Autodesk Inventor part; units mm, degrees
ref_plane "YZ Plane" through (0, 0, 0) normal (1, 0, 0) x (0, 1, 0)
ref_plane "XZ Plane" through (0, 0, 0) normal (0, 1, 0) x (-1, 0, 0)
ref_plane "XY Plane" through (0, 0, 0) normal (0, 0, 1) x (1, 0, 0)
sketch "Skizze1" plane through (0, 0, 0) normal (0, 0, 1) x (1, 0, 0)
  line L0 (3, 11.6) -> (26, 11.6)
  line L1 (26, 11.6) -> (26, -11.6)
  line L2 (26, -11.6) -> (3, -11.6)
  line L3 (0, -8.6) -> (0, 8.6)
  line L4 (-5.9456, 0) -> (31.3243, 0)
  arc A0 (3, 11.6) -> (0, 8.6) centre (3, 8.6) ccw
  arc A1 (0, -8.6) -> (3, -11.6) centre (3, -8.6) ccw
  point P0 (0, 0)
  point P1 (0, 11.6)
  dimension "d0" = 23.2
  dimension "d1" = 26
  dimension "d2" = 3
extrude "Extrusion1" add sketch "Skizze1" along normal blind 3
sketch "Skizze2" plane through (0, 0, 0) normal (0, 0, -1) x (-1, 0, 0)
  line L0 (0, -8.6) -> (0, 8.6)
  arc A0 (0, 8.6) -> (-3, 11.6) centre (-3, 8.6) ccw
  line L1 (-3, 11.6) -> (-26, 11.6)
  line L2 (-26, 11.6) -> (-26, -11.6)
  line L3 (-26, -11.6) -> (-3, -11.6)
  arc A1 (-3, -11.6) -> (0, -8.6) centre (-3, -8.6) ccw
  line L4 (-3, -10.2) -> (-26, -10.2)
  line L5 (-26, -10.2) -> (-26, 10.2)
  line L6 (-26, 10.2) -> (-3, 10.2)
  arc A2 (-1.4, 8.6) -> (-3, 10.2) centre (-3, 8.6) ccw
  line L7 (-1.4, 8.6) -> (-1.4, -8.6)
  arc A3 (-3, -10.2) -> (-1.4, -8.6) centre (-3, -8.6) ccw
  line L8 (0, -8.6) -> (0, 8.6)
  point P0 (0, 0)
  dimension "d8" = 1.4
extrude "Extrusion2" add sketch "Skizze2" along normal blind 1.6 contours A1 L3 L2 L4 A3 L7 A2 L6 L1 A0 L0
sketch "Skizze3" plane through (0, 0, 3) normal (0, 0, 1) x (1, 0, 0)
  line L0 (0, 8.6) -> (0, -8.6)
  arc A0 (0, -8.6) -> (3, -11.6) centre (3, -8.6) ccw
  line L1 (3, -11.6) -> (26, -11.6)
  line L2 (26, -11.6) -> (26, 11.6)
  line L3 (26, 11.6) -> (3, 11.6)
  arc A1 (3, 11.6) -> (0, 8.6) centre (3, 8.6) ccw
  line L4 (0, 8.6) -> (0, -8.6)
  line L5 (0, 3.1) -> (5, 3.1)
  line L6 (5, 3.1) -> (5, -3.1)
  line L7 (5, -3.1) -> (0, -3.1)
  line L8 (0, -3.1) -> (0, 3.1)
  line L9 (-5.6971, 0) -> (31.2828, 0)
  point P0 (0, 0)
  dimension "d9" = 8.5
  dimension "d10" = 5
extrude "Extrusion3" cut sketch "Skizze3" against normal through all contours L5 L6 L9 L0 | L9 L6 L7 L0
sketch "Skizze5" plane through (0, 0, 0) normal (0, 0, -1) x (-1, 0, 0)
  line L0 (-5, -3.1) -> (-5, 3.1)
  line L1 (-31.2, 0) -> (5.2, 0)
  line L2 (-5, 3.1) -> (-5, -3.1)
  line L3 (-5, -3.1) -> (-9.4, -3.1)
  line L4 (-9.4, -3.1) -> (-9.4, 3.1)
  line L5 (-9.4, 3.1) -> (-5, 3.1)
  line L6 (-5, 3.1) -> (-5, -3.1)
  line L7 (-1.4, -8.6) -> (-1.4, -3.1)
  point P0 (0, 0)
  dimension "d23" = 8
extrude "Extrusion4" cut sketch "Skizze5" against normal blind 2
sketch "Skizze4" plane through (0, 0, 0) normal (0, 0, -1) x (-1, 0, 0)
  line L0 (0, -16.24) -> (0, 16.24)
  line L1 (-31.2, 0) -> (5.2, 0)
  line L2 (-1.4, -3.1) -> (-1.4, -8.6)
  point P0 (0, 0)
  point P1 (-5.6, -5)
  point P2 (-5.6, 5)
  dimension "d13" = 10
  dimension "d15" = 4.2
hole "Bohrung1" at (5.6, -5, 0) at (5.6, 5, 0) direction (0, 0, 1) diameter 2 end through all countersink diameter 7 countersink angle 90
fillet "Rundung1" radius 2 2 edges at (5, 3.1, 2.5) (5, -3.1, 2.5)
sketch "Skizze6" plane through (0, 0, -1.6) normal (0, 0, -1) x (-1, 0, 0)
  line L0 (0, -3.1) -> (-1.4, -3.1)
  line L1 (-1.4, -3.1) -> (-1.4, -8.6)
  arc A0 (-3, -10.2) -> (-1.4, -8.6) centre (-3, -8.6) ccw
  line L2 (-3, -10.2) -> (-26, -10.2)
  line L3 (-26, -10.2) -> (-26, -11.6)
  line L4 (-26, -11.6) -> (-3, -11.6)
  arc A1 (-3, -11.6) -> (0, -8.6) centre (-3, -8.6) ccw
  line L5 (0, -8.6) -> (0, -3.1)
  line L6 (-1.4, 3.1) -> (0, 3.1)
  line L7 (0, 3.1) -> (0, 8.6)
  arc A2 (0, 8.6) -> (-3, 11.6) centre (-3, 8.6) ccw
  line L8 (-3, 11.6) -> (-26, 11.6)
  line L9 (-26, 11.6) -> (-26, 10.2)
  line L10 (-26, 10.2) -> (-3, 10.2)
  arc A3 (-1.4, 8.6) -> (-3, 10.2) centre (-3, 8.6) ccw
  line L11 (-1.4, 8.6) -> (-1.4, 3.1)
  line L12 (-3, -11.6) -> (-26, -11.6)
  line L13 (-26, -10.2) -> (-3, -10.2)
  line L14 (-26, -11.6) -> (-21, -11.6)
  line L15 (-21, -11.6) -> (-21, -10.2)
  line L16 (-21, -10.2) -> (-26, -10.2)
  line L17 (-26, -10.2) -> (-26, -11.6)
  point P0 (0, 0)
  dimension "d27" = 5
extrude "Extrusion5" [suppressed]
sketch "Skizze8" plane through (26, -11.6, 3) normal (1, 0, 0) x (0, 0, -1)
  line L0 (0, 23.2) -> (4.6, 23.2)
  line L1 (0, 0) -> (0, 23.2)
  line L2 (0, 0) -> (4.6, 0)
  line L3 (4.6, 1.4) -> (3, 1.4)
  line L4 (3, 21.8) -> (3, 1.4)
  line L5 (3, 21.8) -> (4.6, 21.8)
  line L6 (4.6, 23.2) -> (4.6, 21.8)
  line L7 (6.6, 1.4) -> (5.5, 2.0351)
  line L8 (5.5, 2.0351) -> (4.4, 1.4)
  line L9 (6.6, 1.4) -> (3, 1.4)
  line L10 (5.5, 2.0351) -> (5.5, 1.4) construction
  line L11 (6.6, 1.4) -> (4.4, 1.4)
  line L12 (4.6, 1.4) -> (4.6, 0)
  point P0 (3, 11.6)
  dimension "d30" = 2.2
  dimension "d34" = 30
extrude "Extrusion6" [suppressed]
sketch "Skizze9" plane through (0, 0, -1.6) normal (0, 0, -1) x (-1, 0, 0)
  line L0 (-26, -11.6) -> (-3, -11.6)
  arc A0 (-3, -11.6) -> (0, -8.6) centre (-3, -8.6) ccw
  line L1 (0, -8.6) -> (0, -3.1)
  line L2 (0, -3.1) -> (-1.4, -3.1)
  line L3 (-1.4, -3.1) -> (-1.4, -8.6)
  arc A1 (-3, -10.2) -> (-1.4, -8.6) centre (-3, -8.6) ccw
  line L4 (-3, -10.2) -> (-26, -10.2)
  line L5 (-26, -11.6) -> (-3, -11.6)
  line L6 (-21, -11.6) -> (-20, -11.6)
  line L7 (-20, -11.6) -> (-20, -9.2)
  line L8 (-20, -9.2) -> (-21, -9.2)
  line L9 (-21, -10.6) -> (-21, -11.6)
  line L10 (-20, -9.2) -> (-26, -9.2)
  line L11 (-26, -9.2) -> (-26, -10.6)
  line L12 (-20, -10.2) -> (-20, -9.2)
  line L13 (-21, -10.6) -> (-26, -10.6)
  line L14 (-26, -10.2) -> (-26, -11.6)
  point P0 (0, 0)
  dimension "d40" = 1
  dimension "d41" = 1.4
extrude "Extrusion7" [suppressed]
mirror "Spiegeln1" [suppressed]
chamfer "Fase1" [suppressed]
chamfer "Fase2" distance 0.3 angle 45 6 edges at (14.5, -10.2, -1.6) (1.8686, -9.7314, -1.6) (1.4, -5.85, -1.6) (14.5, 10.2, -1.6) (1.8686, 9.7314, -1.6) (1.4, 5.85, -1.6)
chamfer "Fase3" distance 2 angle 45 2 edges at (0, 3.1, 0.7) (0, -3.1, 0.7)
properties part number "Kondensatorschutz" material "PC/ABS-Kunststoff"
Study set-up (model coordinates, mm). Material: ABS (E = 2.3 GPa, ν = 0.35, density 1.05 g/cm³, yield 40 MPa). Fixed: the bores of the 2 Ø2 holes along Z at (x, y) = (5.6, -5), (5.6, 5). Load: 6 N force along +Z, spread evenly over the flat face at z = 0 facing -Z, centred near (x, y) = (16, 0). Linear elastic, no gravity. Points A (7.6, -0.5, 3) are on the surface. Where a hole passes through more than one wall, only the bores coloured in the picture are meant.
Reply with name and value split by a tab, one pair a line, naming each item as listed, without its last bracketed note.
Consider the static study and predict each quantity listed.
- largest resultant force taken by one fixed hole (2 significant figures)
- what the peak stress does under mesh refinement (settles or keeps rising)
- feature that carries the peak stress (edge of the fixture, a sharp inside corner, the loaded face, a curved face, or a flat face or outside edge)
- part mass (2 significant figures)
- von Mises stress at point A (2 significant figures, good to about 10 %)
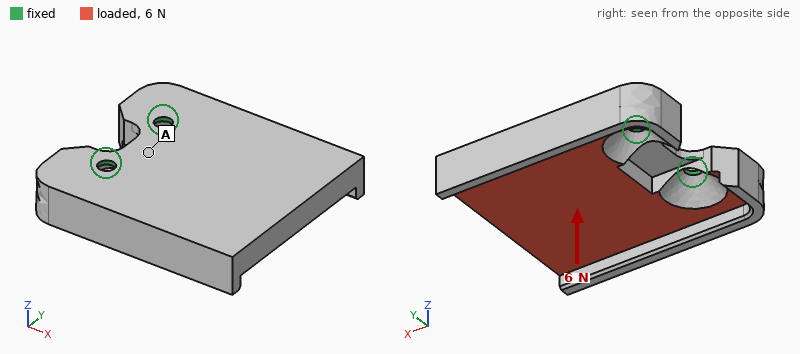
largest resultant force taken by one fixed hole	3.4 N
what the peak stress does under mesh refinement	keeps rising
feature that carries the peak stress	edge of the fixture
part mass	1.8 g
von Mises stress at point A	2.1 MPa
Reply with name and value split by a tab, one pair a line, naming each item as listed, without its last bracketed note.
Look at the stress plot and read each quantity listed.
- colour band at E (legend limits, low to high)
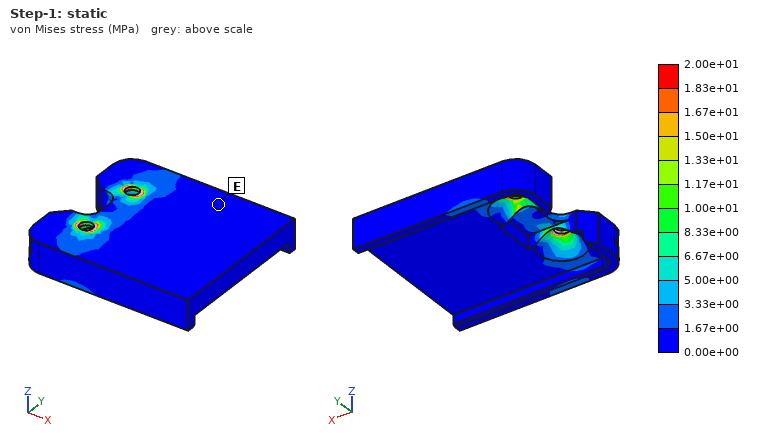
colour band at E	0.00e+00 to 1.67e+00 MPa
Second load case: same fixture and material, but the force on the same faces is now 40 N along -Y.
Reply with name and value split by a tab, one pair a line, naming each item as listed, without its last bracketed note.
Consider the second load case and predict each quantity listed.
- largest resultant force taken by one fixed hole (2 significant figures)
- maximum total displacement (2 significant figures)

largest resultant force taken by one fixed hole	44 N
maximum total displacement	100 µm
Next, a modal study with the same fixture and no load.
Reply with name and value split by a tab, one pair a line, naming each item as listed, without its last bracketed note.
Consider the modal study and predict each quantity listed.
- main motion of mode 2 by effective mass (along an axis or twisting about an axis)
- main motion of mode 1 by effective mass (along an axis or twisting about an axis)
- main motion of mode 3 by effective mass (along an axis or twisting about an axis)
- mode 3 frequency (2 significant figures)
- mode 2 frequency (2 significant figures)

main motion of mode 2 by effective mass	twisting about X
main motion of mode 1 by effective mass	along Z
main motion of mode 3 by effective mass	along Y
mode 3 frequency	3500 Hz
mode 2 frequency	1900 Hz
